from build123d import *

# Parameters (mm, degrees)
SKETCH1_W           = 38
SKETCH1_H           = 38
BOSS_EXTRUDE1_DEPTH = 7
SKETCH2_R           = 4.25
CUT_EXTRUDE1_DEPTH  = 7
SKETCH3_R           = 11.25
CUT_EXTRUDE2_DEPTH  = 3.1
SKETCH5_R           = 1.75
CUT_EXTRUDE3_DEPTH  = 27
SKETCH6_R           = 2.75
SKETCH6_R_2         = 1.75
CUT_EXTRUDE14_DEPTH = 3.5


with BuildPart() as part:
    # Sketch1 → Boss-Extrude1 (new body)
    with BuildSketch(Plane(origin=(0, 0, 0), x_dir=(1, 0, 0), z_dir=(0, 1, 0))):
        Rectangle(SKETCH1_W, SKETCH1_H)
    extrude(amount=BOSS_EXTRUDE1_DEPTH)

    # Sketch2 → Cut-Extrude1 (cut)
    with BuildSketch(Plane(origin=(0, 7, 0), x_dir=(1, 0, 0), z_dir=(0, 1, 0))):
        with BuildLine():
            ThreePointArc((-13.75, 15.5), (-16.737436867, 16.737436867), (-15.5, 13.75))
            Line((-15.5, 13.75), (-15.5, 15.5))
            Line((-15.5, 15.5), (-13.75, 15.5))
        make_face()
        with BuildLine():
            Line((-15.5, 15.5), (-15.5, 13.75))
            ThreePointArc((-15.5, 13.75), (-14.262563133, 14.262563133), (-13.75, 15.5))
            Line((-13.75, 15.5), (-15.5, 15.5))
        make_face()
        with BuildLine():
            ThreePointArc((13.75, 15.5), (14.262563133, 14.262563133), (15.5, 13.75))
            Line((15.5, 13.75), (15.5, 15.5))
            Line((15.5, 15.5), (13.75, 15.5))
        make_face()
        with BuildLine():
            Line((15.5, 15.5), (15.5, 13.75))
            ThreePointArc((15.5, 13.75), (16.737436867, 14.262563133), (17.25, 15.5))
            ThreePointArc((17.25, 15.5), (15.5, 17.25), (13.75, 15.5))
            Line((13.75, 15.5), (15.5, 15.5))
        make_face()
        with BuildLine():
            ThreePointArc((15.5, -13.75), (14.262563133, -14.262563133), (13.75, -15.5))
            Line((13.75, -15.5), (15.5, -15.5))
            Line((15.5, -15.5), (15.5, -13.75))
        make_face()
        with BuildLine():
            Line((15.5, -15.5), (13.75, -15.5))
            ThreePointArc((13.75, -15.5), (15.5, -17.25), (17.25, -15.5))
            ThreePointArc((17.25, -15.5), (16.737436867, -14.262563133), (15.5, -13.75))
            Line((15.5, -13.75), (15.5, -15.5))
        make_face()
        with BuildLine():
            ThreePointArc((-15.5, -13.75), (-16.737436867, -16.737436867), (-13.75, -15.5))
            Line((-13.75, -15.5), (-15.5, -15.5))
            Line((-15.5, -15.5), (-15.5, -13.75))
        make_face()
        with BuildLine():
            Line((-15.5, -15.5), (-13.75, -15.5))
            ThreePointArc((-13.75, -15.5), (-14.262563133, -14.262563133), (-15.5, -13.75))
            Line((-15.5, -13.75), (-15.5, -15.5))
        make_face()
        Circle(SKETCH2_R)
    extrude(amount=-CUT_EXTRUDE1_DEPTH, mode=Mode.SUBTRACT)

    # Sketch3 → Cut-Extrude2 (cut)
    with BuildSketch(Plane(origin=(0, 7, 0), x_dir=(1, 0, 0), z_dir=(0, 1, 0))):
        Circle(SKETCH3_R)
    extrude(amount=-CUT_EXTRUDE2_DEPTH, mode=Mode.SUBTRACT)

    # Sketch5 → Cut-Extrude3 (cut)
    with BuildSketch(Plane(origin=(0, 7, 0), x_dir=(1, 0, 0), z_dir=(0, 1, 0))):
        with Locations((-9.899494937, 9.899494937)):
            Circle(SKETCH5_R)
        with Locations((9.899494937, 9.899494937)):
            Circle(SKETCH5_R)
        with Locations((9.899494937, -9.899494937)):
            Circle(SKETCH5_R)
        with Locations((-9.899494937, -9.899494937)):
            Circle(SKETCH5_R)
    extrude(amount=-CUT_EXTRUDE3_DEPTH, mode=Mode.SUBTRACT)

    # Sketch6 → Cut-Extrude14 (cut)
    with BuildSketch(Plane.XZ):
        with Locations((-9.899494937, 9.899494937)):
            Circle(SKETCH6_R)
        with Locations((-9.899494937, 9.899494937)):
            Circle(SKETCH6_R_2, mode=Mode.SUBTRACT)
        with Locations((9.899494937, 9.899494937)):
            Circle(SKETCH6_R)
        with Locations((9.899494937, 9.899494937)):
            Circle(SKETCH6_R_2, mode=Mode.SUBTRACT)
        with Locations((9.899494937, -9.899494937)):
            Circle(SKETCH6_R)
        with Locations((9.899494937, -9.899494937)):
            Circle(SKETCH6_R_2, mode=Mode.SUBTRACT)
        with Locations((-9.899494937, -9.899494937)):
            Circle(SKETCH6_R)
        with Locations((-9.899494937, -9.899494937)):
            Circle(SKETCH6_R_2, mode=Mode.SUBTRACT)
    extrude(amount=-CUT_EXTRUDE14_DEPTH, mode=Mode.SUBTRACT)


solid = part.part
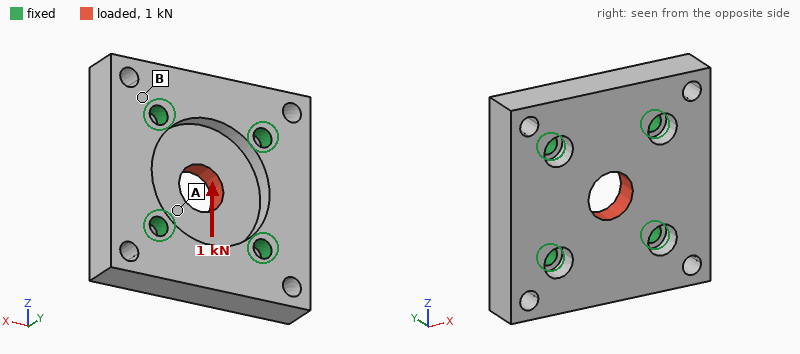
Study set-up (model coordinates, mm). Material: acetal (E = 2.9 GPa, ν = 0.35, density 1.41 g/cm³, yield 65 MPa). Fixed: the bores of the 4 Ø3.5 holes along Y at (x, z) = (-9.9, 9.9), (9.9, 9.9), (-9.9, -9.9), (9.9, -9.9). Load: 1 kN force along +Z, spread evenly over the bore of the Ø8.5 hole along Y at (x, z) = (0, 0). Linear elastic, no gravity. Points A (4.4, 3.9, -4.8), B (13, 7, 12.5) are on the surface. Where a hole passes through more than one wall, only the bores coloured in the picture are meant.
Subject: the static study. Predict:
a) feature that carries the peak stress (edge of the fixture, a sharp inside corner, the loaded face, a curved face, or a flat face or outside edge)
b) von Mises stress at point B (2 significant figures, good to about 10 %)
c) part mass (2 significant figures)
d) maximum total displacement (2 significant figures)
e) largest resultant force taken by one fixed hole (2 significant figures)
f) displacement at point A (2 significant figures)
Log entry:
edge of the fixture
3.6 MPa
11 g
58 µm
260 N
40 µm
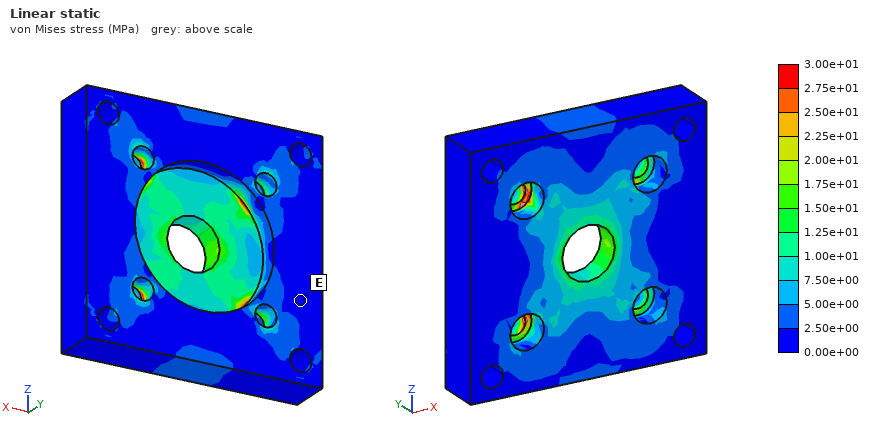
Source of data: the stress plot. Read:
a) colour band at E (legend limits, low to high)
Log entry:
0.00e+00 to 2.50e+00 MPa
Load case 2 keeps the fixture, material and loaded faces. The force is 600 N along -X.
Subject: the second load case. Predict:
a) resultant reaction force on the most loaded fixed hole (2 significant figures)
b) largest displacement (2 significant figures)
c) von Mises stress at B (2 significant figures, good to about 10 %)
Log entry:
150 N
35 µm
1.9 MPa
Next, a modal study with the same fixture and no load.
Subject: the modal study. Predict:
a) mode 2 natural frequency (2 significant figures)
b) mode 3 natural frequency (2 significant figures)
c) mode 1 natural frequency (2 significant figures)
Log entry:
8000 Hz
8000 Hz
7900 Hz
